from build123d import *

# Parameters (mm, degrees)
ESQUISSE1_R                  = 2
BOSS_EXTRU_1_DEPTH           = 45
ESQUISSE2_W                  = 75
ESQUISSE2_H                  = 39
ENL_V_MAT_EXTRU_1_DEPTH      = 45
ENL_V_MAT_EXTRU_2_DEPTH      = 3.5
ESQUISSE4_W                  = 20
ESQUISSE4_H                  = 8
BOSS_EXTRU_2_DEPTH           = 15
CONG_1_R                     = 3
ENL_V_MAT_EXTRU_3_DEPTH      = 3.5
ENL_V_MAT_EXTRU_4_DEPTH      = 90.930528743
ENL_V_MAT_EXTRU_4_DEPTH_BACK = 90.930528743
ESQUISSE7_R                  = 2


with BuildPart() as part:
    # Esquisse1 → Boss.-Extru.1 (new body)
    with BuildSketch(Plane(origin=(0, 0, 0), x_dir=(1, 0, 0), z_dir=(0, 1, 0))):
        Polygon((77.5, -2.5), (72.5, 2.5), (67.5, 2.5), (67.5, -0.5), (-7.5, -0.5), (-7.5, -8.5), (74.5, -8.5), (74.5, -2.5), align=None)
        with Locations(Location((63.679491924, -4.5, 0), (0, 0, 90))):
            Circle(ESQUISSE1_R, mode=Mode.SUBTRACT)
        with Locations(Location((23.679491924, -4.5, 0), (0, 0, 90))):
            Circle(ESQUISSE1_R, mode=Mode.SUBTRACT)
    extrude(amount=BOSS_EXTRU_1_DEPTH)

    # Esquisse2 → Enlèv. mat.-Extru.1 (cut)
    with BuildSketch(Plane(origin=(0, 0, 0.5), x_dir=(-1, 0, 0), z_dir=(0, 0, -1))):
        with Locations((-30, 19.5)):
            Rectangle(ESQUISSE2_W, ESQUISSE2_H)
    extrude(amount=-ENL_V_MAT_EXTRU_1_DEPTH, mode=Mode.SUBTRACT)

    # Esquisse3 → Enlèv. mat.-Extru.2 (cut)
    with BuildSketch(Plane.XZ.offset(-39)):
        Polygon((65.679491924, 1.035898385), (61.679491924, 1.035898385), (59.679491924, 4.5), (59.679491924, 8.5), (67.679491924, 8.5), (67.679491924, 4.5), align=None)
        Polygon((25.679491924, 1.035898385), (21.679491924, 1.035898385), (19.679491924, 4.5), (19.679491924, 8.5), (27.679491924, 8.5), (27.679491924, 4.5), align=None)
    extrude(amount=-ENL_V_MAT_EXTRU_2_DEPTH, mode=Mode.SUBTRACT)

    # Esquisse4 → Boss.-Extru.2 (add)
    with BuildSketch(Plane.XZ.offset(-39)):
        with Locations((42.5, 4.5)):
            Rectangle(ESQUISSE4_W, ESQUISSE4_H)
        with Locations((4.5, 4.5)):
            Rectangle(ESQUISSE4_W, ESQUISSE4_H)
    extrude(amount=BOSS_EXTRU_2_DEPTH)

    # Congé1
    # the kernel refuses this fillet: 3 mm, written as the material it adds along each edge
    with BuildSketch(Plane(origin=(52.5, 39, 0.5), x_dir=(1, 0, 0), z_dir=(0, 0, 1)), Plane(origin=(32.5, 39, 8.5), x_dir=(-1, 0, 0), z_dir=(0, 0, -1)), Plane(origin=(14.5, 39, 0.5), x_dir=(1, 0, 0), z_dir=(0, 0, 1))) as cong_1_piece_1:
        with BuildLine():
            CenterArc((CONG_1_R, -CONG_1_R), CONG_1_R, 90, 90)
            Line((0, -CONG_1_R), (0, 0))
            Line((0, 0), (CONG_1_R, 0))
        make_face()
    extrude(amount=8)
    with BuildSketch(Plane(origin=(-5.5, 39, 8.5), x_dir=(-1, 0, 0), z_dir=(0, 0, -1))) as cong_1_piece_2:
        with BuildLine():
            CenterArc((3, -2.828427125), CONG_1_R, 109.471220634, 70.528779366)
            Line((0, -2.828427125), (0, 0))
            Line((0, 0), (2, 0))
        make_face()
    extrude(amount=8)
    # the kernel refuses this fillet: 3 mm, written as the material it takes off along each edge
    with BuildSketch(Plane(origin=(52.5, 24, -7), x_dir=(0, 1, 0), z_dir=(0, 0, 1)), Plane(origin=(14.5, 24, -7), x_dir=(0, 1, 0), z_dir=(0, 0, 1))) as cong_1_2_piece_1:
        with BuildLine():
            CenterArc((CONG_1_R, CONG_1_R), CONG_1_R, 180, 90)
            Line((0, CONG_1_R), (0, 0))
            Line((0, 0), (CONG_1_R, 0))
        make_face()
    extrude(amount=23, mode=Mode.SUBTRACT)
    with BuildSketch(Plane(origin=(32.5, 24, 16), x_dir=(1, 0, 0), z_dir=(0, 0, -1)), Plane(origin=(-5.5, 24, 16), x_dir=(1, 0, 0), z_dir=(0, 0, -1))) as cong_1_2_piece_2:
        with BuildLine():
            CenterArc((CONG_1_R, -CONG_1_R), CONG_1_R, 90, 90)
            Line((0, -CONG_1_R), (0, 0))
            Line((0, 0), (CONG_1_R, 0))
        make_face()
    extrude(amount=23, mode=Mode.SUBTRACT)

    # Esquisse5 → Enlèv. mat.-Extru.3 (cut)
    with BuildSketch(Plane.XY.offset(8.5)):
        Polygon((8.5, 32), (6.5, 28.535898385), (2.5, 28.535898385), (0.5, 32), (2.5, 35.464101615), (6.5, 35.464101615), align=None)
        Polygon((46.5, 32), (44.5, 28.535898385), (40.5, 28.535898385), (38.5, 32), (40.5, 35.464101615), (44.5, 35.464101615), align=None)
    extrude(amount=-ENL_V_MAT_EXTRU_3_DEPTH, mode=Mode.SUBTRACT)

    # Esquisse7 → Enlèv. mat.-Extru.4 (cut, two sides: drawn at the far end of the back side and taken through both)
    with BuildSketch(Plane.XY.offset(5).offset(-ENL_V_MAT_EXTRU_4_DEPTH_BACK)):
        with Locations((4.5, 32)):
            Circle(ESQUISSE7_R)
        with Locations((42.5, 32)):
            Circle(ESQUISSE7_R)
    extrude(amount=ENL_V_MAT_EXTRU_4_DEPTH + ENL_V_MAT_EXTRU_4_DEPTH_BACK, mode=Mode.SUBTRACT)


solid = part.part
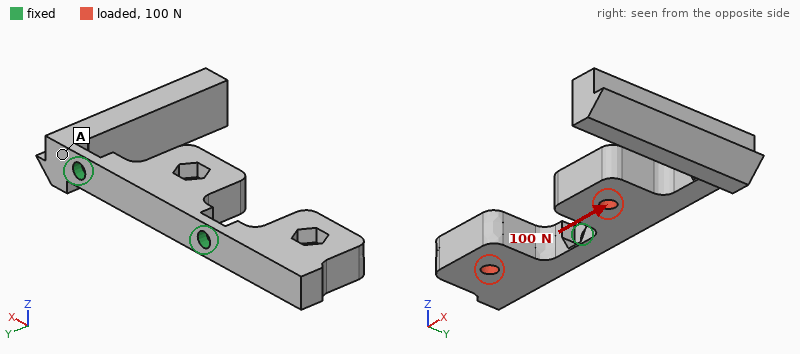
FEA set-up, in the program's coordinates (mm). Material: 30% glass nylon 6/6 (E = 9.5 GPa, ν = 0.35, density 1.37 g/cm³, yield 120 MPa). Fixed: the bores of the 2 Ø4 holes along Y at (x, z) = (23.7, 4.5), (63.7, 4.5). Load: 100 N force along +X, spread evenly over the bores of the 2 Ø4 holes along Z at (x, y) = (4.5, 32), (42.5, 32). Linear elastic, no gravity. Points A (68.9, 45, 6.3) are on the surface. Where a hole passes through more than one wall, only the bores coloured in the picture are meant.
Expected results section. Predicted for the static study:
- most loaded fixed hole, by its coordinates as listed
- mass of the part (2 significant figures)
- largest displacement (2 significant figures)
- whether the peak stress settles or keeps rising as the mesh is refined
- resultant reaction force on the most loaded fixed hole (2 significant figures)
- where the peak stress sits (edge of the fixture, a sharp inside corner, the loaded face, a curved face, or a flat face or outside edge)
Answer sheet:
(23.7, 4.5)
15 g
0.40 mm
keeps rising
61 N
a sharp inside corner
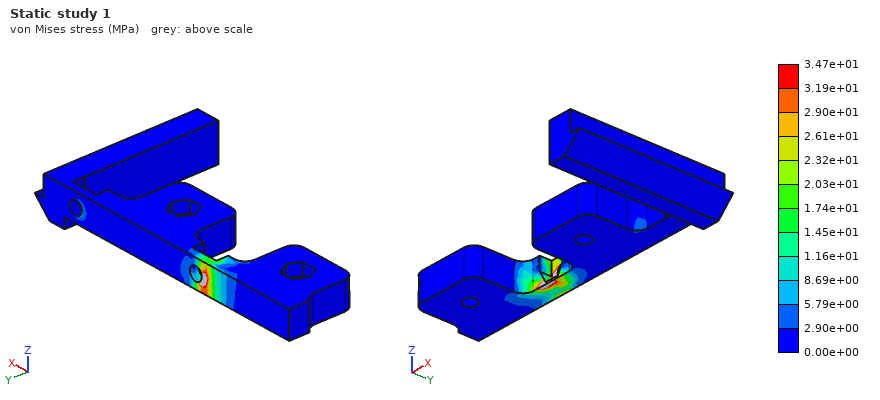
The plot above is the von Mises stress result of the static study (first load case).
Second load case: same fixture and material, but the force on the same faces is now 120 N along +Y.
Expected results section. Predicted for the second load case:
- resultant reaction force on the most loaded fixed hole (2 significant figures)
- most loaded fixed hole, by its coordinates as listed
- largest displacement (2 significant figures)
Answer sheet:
98 N
(23.7, 4.5)
0.69 mm
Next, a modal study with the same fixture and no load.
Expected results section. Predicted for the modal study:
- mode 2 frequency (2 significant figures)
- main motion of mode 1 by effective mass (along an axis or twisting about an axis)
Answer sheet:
770 Hz
along X
